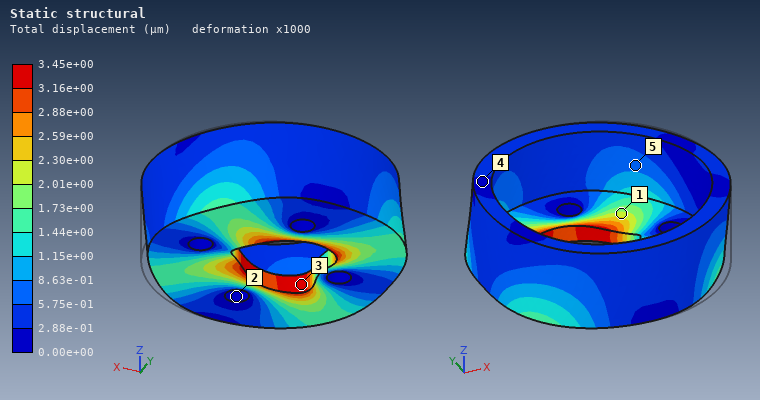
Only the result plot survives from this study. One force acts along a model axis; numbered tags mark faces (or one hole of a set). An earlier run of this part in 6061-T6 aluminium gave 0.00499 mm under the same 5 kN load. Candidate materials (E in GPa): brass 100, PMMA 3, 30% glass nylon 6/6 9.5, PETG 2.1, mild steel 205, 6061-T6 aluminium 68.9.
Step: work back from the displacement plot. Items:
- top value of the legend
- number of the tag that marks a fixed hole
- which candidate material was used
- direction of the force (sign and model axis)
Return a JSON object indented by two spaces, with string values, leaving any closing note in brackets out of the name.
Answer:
{
  "top value of the legend": "3.45e+00 µm",
  "number of the tag that marks a fixed hole": "2",
  "which candidate material was used": "brass",
  "direction of the force": "-X"
}
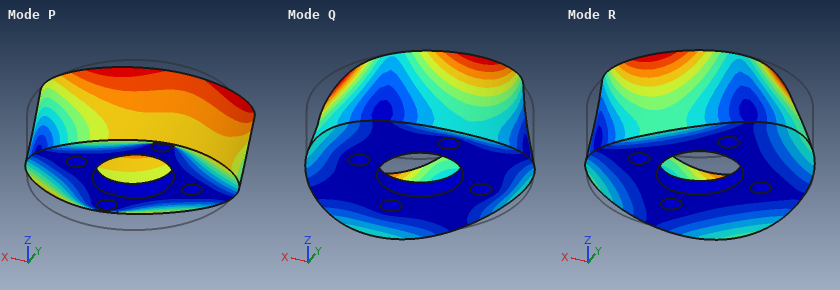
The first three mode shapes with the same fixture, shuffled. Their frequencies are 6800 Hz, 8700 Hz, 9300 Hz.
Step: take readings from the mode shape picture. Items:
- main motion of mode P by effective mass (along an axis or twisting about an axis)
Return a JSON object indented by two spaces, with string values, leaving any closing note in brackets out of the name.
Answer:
{
  "main motion of mode P by effective mass": "along Y"
}
